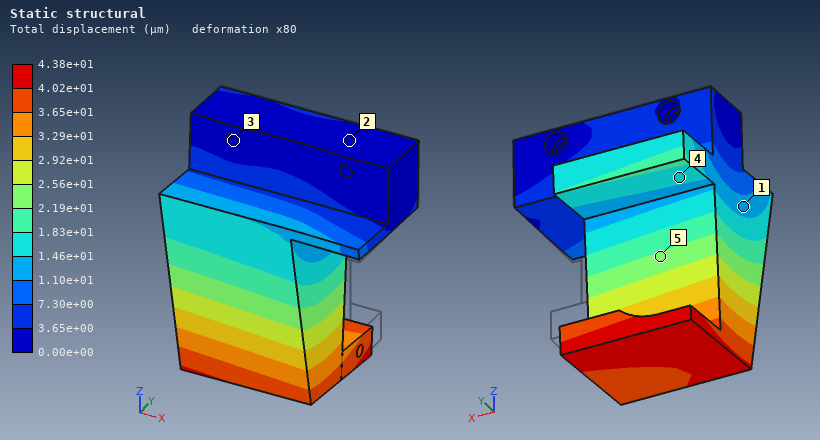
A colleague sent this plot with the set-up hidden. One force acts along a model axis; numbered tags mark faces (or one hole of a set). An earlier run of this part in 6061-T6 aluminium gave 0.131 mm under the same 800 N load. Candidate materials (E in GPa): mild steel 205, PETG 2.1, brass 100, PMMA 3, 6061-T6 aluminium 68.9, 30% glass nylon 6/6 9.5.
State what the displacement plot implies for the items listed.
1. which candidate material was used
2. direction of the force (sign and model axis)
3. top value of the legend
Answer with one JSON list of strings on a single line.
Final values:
["mild steel", "-Y", "4.38e+01 µm"]
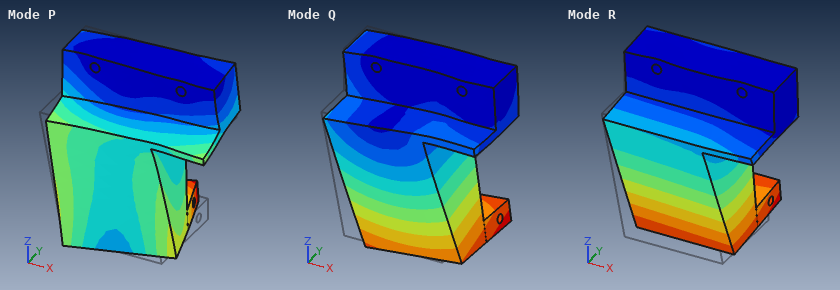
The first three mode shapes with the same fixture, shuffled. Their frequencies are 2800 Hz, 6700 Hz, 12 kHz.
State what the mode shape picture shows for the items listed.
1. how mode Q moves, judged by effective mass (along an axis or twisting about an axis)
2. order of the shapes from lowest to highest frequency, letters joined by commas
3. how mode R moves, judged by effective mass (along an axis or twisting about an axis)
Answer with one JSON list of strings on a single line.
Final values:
["along X", "R, Q, P", "along Y"]
